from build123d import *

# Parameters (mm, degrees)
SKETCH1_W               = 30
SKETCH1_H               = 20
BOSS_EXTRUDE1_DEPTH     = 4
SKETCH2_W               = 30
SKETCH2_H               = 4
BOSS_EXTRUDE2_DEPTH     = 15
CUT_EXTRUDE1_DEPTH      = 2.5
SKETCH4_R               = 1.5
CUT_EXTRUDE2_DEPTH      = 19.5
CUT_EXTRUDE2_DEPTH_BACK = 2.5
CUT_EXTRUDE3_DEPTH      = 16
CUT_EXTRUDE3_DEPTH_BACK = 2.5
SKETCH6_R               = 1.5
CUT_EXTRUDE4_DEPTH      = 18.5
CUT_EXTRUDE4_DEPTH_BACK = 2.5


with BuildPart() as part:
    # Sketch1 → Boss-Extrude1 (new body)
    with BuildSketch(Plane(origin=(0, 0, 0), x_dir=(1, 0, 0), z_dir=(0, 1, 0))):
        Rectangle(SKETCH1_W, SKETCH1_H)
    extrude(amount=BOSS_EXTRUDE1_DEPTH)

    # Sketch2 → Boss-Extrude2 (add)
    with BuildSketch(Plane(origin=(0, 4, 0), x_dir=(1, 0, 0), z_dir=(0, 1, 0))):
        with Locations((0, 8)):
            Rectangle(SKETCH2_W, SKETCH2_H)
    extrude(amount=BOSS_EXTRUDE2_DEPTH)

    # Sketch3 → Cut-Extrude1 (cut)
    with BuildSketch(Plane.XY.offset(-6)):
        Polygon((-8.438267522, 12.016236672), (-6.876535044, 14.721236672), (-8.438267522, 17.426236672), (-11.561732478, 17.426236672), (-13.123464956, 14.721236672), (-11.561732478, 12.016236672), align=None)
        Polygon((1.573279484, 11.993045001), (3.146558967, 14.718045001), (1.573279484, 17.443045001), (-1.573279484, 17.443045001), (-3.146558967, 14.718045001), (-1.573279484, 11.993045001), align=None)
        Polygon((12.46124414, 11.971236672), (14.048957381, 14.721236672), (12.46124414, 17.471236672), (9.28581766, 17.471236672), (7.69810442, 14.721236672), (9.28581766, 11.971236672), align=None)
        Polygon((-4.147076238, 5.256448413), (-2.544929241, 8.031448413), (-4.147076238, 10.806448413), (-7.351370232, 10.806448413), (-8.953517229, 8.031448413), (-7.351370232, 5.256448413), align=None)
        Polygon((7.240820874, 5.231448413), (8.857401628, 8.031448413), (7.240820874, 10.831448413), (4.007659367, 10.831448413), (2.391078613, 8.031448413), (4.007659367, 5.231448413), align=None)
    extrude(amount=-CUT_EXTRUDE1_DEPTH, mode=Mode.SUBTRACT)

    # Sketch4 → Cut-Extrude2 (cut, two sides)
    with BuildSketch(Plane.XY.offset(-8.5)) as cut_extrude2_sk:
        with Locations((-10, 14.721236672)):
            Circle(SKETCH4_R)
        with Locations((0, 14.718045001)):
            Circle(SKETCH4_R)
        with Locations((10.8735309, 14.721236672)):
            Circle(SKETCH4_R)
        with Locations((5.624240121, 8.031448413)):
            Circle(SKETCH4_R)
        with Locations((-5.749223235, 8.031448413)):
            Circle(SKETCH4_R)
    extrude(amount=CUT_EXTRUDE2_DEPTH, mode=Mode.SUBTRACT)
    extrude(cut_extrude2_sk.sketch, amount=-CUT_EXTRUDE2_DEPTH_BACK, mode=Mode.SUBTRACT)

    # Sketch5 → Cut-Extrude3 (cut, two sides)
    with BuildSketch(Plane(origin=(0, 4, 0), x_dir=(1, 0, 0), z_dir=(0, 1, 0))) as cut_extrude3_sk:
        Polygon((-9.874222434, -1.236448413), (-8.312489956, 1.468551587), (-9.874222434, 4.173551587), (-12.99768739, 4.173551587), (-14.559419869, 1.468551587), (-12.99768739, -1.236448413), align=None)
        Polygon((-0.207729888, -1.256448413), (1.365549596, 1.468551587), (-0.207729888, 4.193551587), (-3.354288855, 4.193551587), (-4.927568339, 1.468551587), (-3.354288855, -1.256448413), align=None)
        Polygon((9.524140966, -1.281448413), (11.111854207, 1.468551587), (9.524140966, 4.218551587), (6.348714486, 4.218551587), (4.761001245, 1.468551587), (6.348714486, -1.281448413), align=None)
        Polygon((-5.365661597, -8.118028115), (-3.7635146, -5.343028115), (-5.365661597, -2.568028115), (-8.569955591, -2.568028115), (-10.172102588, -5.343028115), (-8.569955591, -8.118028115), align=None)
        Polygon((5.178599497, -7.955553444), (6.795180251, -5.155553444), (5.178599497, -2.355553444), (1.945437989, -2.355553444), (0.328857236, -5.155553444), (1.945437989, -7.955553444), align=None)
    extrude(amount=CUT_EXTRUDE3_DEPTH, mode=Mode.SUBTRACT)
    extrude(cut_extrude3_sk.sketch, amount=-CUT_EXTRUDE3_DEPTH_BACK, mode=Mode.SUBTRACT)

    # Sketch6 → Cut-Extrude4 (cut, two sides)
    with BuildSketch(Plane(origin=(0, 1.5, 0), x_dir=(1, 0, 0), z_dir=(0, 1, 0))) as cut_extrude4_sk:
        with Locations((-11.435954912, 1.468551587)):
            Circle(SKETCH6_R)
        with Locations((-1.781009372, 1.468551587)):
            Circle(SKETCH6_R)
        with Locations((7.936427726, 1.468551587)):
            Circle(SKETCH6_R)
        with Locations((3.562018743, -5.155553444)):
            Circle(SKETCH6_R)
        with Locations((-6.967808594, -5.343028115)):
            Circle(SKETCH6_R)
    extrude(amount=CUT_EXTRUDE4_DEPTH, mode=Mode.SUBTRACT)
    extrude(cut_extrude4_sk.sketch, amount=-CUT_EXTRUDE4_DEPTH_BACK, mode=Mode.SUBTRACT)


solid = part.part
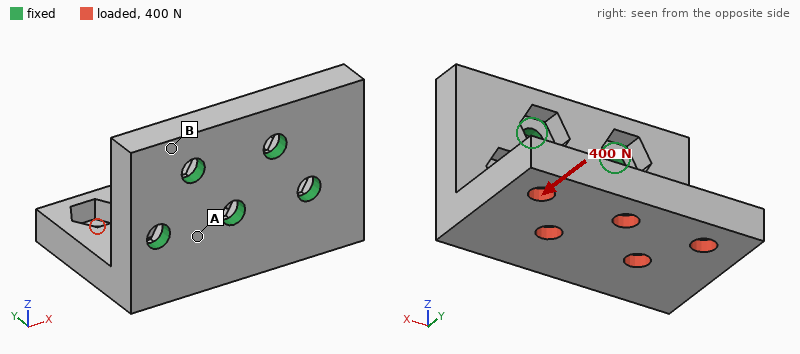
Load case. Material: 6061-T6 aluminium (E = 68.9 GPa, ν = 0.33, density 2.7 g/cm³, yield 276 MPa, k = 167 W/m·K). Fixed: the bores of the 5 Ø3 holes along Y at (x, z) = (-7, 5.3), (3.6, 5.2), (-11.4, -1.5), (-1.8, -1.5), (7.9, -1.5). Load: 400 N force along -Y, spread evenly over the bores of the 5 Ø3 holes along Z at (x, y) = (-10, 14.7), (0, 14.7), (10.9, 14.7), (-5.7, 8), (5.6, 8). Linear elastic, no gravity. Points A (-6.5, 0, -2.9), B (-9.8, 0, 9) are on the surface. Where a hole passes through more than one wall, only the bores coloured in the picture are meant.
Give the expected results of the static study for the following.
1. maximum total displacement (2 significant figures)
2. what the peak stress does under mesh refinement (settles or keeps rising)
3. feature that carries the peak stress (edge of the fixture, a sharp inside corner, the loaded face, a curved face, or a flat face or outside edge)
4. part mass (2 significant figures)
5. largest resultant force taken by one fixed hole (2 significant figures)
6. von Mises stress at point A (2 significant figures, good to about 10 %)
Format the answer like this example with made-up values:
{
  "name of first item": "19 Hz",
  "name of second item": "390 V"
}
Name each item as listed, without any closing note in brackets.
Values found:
{
  "maximum total displacement": "49 µm",
  "what the peak stress does under mesh refinement": "keeps rising",
  "feature that carries the peak stress": "edge of the fixture",
  "part mass": "9.3 g",
  "largest resultant force taken by one fixed hole": "260 N",
  "von Mises stress at point A": "30 MPa"
}
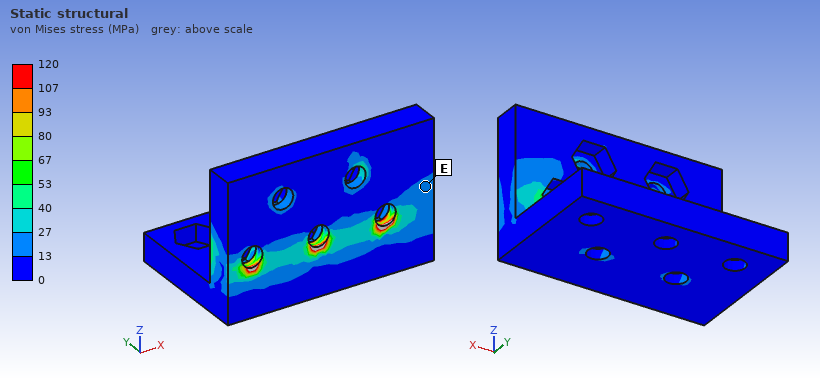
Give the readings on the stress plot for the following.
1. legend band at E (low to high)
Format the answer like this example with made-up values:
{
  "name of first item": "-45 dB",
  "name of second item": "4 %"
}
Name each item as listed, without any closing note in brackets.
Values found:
{
  "legend band at E": "13 to 27 MPa"
}
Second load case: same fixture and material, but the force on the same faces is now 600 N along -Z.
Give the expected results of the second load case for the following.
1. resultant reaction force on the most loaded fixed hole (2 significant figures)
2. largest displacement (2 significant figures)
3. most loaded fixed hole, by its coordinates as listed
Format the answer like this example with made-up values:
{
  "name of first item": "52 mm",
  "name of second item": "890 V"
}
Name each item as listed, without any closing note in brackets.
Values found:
{
  "resultant reaction force on the most loaded fixed hole": "510 N",
  "largest displacement": "0.16 mm",
  "most loaded fixed hole, by its coordinates as listed": "(3.6, 5.2)"
}
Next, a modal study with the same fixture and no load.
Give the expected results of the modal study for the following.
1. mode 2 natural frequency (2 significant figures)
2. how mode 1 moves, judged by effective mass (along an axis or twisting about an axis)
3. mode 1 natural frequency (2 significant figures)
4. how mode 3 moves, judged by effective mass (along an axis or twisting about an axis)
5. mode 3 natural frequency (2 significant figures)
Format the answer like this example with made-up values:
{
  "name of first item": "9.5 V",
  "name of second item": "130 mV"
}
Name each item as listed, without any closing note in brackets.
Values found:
{
  "mode 2 natural frequency": "11 kHz",
  "how mode 1 moves, judged by effective mass": "along Z",
  "mode 1 natural frequency": "5900 Hz",
  "how mode 3 moves, judged by effective mass": "along X",
  "mode 3 natural frequency": "17 kHz"
}
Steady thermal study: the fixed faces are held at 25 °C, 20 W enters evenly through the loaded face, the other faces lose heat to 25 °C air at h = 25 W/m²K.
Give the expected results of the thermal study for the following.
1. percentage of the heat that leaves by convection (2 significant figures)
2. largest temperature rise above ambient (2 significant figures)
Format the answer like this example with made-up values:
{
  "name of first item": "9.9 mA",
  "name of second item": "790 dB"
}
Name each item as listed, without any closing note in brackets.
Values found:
{
  "percentage of the heat that leaves by convection": "3.5 %",
  "largest temperature rise above ambient": "23 K"
}
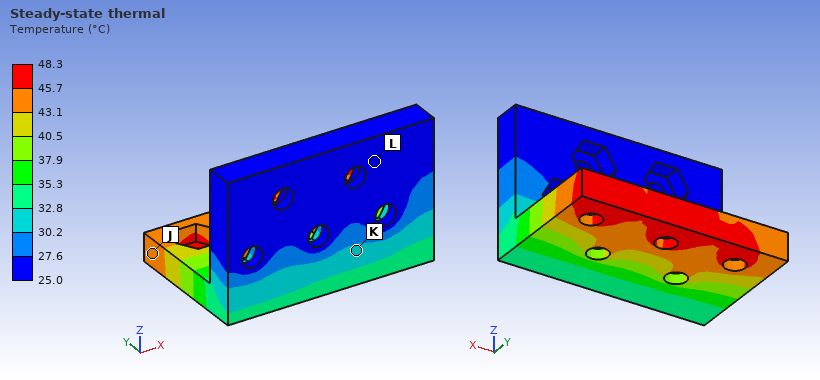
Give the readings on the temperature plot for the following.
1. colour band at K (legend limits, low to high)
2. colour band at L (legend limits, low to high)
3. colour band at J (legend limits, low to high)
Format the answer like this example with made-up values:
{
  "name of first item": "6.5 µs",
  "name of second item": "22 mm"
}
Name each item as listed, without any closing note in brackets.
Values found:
{
  "colour band at K": "30.2 to 32.8 °C",
  "colour band at L": "25.0 to 27.6 °C",
  "colour band at J": "43.1 to 45.7 °C"
}
